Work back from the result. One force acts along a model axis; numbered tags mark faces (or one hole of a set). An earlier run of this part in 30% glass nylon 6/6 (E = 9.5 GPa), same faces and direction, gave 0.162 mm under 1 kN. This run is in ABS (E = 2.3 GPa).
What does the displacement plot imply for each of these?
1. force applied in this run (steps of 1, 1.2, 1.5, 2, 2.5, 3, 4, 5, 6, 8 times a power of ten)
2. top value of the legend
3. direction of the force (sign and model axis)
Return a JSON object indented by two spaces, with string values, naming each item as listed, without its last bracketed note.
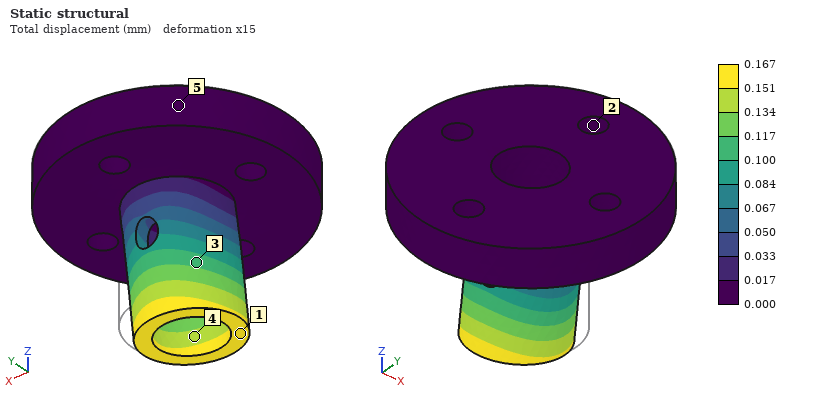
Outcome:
{
  "force applied in this run": "250 N",
  "top value of the legend": "0.167 mm",
  "direction of the force": "-Y"
}
